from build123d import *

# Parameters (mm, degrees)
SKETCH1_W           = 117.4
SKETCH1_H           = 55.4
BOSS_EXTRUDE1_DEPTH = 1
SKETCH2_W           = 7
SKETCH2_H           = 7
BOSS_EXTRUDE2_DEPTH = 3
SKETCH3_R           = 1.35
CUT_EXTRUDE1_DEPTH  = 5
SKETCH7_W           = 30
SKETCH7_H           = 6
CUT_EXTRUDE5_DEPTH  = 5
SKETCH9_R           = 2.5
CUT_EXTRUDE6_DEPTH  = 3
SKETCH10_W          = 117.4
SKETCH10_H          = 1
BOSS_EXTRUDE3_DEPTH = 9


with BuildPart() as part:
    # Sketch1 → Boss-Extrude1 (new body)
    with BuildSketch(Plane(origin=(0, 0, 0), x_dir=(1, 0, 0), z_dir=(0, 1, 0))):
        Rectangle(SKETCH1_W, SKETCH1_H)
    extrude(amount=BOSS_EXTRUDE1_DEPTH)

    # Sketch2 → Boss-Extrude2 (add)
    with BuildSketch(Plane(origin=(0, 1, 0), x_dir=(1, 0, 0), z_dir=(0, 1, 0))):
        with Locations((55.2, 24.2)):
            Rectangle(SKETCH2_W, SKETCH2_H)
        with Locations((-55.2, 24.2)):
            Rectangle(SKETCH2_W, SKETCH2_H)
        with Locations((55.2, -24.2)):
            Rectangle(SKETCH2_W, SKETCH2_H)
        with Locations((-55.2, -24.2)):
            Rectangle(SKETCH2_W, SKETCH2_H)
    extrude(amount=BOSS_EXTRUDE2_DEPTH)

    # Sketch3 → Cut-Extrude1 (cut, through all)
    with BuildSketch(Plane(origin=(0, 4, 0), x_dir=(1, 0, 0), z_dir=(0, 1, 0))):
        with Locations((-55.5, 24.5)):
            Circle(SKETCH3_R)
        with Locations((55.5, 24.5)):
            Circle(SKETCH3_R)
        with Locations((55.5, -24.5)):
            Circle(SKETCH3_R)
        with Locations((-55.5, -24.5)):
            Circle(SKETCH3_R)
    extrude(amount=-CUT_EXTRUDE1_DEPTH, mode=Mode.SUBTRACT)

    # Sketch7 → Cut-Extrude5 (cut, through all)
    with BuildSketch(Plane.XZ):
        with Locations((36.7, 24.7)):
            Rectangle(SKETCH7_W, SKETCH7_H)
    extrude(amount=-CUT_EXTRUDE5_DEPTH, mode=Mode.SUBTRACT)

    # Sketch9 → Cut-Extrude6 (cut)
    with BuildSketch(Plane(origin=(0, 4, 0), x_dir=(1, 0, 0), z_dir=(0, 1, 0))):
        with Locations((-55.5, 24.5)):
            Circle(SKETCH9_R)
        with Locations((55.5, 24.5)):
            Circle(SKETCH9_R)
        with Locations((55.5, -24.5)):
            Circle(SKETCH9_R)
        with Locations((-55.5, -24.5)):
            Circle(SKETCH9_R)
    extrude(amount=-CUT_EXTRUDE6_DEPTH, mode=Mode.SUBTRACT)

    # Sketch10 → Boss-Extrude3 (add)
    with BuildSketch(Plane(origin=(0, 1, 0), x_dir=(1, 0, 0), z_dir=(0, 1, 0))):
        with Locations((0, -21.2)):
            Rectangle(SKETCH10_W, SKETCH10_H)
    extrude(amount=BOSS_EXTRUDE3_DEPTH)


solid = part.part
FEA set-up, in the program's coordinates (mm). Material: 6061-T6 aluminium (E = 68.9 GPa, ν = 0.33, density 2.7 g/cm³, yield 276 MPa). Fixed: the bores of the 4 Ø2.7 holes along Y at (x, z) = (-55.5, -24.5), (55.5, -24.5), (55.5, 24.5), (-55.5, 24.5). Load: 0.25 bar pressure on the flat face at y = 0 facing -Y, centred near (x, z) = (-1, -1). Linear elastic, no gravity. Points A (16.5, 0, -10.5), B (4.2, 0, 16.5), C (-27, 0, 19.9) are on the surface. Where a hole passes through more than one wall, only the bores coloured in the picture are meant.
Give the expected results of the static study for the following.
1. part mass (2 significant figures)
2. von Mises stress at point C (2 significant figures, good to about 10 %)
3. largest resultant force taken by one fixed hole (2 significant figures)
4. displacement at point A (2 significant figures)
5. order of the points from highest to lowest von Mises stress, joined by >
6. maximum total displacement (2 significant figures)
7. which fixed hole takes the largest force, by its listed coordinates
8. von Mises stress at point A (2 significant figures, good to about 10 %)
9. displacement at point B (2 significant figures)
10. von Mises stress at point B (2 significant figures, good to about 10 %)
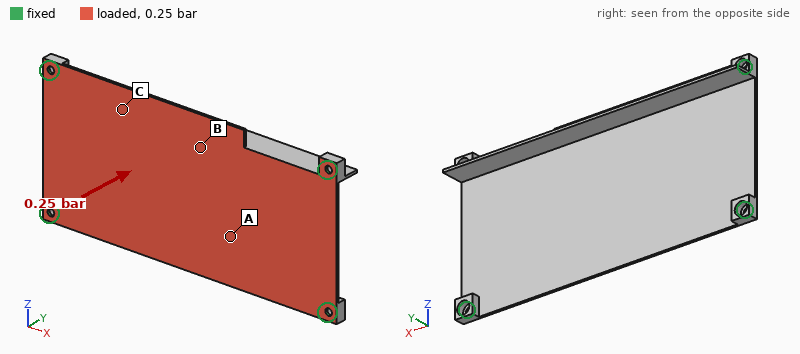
21 g
27 MPa
78 N
0.85 mm
A > C > B
1.4 mm
(-55.5, 24.5)
42 MPa
0.23 mm
13 MPa
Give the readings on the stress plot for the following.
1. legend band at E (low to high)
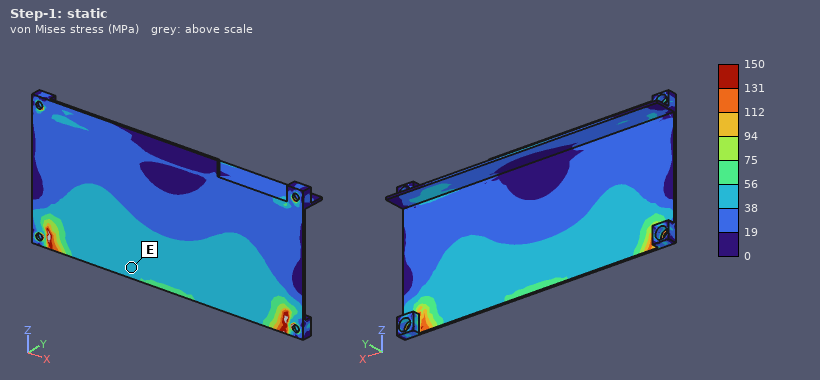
38 to 56 MPa
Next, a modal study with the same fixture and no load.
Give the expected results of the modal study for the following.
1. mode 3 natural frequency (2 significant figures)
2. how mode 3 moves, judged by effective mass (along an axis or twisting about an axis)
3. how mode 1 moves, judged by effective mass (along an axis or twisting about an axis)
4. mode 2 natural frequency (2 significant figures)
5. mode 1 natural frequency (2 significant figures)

1600 Hz
along Y
along Y
1400 Hz
550 Hz
